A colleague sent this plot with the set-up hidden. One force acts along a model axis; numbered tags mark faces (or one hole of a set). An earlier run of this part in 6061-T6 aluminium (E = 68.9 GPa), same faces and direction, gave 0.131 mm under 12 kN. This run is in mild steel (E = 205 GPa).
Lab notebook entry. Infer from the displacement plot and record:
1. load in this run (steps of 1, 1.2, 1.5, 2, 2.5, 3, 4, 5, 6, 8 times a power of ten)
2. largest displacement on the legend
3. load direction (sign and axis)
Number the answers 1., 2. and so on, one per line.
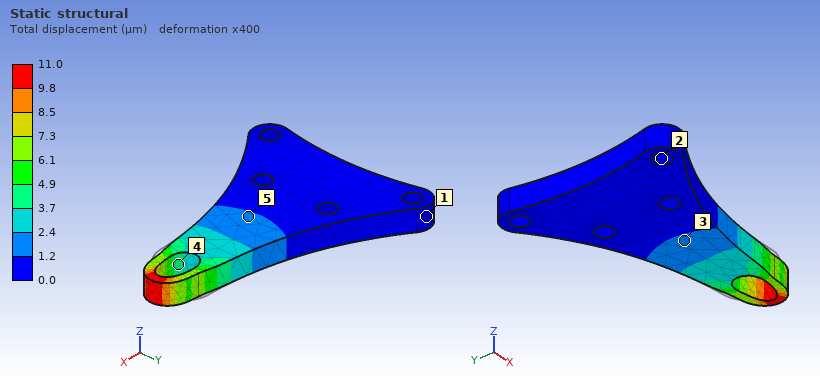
1. 3 kN
2. 11.0 µm
3. +X
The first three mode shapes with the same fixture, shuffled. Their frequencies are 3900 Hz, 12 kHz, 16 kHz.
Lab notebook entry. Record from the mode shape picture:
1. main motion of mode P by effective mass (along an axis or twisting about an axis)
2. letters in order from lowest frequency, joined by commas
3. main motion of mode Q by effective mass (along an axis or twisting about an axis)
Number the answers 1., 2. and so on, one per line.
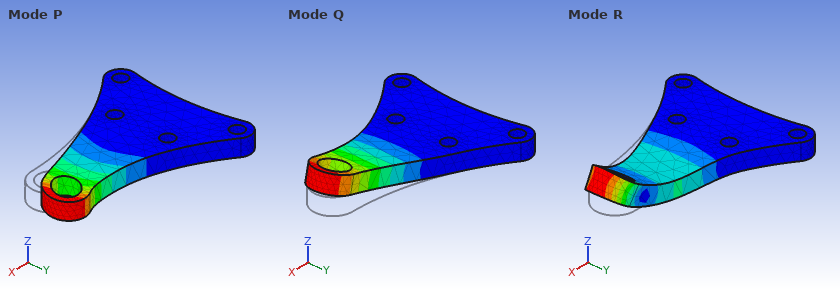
1. along Y
2. Q, P, R
3. along Z
